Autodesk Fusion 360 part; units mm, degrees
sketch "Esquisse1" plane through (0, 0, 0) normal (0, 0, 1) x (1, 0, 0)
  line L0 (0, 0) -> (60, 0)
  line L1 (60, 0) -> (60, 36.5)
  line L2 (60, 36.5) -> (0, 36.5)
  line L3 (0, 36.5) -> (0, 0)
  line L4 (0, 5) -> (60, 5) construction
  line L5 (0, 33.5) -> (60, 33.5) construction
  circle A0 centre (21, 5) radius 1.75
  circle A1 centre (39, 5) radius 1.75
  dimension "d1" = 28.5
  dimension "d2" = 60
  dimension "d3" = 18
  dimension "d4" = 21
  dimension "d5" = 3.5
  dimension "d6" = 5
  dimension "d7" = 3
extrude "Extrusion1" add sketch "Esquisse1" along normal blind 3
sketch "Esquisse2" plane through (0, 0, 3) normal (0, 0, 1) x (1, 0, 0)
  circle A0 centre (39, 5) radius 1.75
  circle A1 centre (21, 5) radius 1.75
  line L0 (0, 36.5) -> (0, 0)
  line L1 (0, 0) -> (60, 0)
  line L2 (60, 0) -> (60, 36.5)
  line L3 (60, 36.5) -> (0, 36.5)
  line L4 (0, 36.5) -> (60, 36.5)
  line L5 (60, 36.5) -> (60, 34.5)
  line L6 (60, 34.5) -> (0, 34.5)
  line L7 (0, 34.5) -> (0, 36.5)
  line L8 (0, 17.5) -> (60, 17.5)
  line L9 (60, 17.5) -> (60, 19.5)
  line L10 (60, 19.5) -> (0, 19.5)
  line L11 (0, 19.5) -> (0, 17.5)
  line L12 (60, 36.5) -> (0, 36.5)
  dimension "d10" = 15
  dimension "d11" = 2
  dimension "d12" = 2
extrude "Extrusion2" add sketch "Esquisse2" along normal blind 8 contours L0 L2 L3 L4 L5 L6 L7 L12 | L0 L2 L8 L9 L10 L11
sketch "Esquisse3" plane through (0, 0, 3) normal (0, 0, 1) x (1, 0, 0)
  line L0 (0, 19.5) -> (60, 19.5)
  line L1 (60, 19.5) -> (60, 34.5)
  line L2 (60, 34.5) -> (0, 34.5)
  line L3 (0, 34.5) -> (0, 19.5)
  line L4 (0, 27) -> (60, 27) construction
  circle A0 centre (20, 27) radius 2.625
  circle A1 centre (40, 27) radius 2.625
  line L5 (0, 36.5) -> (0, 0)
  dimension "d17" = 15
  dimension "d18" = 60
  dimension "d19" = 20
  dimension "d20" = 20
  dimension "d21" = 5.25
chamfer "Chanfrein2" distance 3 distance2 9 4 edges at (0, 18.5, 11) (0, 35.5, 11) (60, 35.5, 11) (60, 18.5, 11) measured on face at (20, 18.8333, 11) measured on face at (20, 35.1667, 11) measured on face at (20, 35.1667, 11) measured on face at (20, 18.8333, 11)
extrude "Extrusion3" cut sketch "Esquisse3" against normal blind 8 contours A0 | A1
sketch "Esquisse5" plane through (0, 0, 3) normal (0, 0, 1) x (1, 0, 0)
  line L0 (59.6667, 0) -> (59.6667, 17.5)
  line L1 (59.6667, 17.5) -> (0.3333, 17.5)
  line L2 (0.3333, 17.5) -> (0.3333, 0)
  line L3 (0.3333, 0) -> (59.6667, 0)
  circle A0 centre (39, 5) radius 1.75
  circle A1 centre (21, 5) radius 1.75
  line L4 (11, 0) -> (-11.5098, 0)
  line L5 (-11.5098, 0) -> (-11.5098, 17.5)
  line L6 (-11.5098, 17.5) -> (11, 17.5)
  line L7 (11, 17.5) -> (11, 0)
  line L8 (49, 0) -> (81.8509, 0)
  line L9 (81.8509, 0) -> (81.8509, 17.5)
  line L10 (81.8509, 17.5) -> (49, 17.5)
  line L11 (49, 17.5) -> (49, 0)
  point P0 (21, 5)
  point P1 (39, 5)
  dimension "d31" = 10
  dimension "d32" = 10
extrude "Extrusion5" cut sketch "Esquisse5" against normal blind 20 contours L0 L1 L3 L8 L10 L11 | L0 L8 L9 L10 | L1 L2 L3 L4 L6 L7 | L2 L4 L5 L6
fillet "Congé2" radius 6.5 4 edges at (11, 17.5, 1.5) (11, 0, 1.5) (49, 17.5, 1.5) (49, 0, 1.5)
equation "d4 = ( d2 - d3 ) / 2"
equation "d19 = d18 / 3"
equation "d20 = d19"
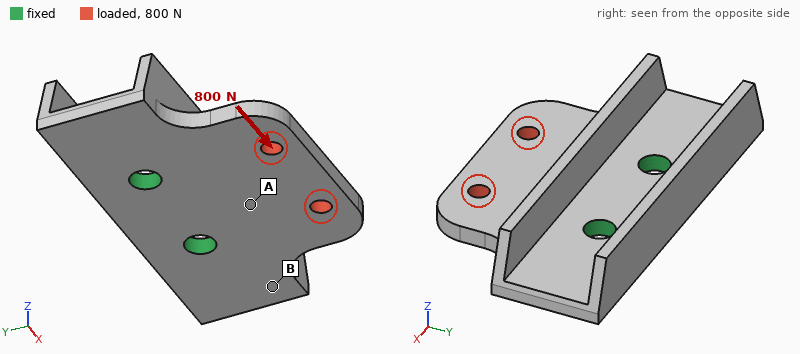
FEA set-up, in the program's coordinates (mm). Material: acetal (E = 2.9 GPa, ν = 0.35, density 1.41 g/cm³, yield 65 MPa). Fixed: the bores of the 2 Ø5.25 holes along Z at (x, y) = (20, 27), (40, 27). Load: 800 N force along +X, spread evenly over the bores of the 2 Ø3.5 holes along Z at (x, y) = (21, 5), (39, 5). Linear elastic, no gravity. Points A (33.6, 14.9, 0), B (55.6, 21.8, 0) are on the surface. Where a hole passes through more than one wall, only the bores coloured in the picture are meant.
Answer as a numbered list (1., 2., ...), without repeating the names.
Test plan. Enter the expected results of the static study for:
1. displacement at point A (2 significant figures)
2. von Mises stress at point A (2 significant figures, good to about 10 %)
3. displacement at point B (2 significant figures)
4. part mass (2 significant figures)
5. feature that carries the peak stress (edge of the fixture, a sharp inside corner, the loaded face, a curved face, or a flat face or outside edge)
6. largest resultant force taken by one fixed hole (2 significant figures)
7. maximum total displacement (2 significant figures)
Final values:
1. 0.12 mm
2. 18 MPa
3. 0.16 mm
4. 9.9 g
5. edge of the fixture
6. 810 N
7. 0.31 mm
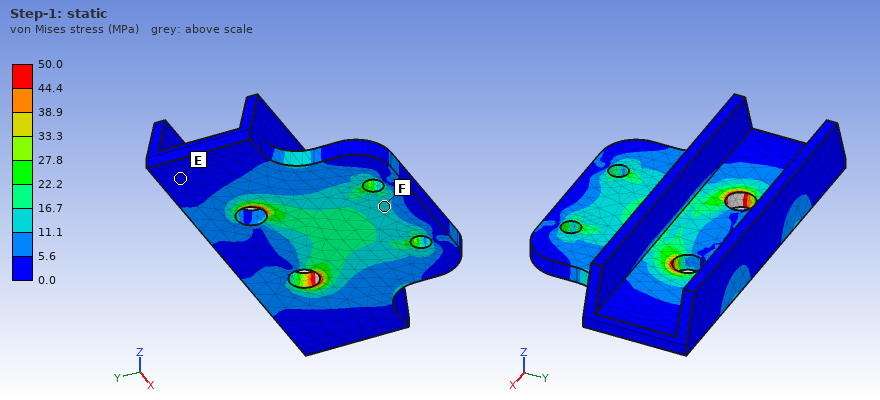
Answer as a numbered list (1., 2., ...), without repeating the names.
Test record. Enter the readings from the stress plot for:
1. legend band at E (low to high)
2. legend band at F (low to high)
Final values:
1. 0.0 to 5.6 MPa
2. 11.1 to 16.7 MPa
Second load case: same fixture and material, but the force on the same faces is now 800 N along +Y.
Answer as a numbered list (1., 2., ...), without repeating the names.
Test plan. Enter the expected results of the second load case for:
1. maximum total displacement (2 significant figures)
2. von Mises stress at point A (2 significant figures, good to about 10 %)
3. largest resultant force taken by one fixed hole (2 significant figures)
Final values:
1. 89 µm
2. 7.0 MPa
3. 410 N
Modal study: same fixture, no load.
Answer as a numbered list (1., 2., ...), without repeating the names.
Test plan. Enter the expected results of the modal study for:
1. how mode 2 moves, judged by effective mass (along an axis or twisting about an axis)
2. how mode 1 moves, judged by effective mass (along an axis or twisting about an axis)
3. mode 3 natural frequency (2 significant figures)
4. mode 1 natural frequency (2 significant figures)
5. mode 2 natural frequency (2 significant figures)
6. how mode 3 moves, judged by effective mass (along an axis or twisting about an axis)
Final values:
1. twisting about Y
2. along Z
3. 2700 Hz
4. 1200 Hz
5. 1900 Hz
6. twisting about Y
